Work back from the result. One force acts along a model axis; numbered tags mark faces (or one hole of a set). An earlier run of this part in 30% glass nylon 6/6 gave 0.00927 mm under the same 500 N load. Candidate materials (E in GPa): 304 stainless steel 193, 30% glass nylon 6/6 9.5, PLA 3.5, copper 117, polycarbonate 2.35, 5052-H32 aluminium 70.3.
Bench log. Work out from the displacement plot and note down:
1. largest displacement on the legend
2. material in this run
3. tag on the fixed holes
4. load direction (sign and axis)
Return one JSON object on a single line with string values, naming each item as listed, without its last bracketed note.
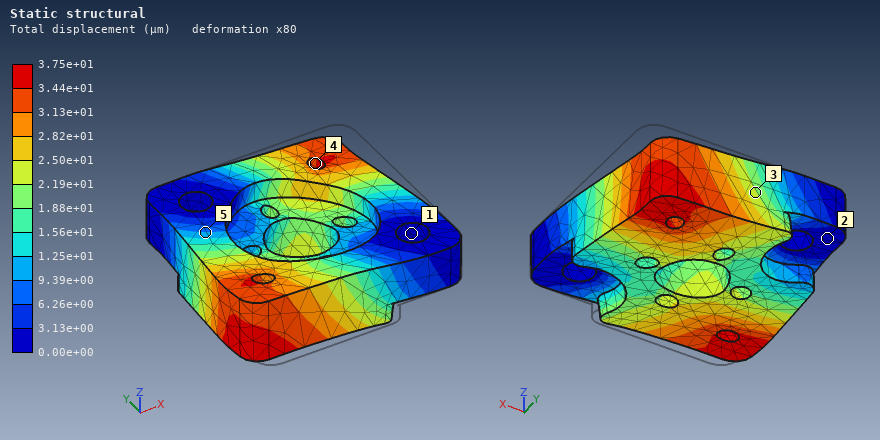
{"largest displacement on the legend": "3.75e+01 µm", "material in this run": "polycarbonate", "tag on the fixed holes": "1", "load direction": "-X"}
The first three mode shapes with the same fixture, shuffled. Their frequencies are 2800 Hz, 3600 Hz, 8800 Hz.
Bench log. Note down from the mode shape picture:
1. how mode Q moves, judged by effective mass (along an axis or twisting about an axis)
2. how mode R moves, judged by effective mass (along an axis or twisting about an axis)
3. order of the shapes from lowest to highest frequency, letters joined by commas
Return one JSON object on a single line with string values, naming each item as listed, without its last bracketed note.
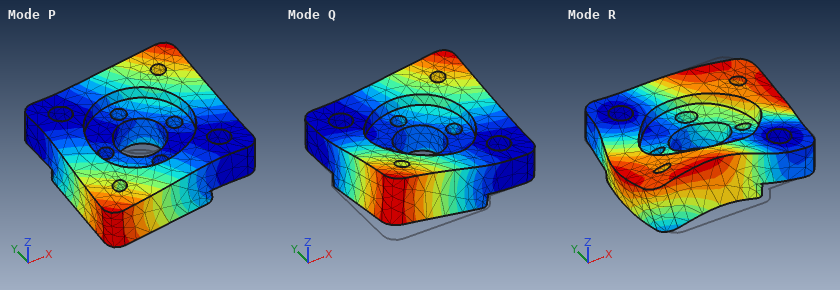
{"how mode Q moves, judged by effective mass": "along Z", "how mode R moves, judged by effective mass": "twisting about Z", "order of the shapes from lowest to highest frequency, letters joined by commas": "P, Q, R"}
